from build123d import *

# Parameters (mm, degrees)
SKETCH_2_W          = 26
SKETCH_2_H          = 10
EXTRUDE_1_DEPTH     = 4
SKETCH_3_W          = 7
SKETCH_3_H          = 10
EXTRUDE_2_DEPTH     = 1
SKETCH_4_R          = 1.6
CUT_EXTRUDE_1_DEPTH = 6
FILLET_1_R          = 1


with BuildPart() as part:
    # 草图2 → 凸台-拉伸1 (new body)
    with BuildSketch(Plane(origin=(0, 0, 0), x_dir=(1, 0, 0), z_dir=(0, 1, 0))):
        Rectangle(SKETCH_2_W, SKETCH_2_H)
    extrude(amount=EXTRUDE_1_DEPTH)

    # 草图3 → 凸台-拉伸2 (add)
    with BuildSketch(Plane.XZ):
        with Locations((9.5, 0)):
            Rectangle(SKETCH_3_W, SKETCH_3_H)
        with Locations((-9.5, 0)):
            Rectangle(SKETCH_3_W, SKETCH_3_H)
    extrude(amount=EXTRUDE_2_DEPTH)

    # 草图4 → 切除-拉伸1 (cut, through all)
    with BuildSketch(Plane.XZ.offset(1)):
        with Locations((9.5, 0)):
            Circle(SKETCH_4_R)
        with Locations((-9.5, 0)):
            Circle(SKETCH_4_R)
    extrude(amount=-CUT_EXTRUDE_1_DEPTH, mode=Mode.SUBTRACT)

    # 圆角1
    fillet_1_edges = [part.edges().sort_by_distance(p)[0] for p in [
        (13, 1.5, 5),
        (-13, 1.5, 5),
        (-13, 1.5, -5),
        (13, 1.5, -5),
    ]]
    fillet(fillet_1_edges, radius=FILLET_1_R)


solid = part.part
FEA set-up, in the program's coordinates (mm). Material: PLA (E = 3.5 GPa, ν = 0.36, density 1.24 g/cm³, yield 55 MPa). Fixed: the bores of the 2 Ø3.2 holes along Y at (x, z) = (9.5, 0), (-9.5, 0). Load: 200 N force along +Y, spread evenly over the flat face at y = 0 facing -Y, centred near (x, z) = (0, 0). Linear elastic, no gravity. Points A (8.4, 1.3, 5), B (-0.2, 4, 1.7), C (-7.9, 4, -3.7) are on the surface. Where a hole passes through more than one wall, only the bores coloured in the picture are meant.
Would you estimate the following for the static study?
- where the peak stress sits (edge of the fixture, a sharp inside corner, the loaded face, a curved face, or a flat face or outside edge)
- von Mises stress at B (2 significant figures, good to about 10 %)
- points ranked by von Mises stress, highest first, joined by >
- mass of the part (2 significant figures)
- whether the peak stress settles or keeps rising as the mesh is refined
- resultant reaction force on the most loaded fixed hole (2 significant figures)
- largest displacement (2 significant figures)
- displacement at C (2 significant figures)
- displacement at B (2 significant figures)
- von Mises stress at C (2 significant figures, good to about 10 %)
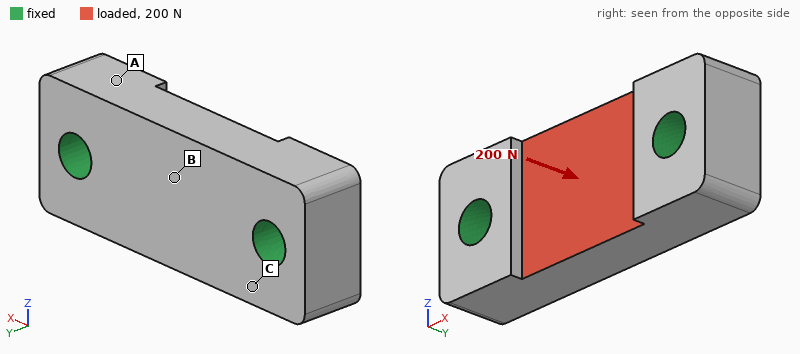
edge of the fixture
7.0 MPa
B > C > A
1.4 g
keeps rising
100 N
32 µm
7.3 µm
27 µm
3.7 MPa
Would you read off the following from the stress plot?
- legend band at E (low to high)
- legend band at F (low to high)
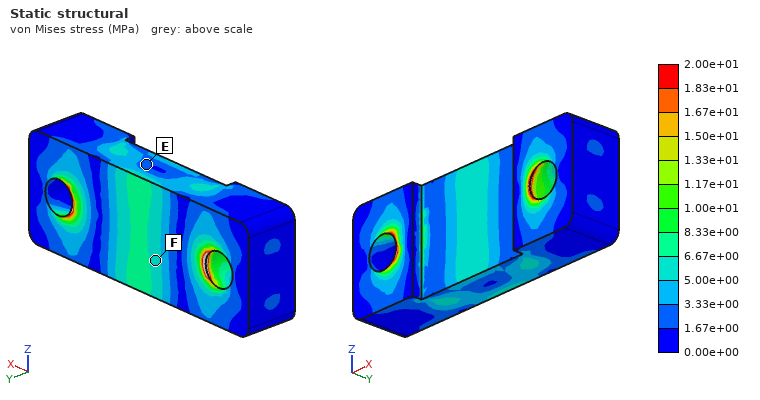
1.67e+00 to 3.33e+00 MPa
5.00e+00 to 6.67e+00 MPa
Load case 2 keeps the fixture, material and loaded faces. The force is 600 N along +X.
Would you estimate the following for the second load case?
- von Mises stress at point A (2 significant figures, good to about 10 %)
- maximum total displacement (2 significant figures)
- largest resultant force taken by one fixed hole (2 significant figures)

4.1 MPa
22 µm
310 N
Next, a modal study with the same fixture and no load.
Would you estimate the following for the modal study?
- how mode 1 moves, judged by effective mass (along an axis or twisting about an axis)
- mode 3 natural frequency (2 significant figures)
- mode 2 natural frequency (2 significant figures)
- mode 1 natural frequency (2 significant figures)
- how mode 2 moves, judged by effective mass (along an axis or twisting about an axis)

along Y
22 kHz
21 kHz
18 kHz
along Z
